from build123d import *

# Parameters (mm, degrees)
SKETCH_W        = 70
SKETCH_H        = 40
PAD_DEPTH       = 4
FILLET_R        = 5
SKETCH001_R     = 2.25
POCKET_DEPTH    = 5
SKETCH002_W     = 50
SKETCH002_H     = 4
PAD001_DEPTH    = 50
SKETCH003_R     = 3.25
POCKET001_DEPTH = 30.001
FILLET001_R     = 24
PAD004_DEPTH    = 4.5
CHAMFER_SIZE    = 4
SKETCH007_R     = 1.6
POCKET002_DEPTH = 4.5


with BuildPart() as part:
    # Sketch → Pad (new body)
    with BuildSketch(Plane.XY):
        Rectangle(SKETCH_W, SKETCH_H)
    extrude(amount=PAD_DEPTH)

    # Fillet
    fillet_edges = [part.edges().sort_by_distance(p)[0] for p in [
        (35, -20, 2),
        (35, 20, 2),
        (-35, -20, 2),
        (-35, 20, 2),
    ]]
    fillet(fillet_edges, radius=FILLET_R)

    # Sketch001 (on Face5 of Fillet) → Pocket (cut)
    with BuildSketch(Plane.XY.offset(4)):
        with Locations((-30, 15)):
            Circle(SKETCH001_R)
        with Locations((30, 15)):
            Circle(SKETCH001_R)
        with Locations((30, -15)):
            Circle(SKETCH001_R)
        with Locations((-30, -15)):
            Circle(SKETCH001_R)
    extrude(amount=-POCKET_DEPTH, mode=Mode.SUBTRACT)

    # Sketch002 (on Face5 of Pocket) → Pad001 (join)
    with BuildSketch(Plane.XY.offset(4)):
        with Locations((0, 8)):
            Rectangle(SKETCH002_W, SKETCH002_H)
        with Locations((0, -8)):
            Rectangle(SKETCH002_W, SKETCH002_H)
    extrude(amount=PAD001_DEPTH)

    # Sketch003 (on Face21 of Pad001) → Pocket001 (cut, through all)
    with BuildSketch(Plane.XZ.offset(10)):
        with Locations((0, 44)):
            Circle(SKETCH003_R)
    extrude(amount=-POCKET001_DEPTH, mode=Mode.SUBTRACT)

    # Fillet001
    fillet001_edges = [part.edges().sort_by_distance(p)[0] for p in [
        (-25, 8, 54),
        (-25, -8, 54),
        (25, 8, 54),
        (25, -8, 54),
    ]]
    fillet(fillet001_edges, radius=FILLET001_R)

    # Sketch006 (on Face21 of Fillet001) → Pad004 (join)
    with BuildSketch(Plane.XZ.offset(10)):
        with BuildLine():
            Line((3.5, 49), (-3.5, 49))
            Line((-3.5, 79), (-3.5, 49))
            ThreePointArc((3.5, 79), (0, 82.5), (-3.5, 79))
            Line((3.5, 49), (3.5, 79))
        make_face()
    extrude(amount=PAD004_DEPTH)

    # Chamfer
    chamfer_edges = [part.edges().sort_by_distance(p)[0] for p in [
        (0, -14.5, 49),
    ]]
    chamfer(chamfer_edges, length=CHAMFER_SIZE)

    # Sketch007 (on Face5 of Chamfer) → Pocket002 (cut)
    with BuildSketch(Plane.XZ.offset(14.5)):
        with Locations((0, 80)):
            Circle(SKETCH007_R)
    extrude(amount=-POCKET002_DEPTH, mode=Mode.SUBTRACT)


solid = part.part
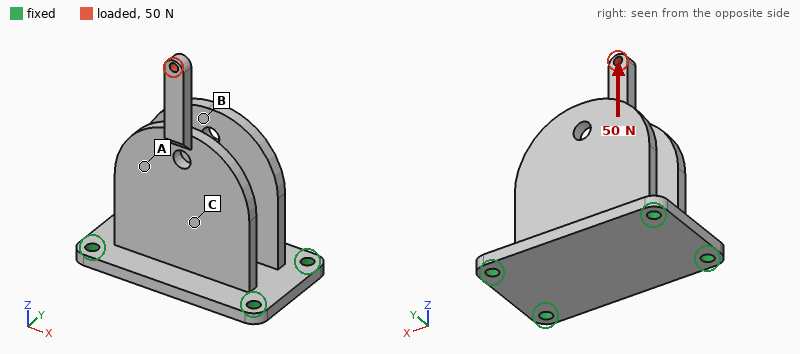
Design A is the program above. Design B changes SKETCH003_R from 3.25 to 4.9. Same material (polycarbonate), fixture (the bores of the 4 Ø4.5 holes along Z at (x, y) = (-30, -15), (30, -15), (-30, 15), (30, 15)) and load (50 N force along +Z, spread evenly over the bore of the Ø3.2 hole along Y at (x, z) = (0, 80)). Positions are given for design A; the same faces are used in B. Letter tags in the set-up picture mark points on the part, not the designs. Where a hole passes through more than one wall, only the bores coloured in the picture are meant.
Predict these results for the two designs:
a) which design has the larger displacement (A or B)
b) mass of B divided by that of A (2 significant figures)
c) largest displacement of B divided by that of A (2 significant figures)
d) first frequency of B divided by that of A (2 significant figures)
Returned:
B
0.99
1.1
1.0
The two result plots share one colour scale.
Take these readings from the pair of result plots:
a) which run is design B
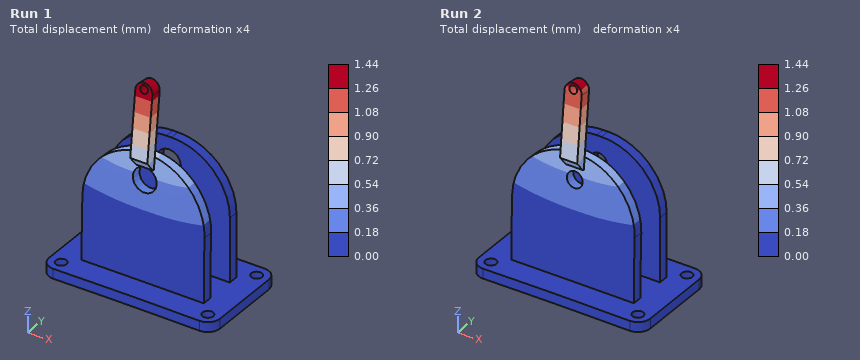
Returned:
Run 1
